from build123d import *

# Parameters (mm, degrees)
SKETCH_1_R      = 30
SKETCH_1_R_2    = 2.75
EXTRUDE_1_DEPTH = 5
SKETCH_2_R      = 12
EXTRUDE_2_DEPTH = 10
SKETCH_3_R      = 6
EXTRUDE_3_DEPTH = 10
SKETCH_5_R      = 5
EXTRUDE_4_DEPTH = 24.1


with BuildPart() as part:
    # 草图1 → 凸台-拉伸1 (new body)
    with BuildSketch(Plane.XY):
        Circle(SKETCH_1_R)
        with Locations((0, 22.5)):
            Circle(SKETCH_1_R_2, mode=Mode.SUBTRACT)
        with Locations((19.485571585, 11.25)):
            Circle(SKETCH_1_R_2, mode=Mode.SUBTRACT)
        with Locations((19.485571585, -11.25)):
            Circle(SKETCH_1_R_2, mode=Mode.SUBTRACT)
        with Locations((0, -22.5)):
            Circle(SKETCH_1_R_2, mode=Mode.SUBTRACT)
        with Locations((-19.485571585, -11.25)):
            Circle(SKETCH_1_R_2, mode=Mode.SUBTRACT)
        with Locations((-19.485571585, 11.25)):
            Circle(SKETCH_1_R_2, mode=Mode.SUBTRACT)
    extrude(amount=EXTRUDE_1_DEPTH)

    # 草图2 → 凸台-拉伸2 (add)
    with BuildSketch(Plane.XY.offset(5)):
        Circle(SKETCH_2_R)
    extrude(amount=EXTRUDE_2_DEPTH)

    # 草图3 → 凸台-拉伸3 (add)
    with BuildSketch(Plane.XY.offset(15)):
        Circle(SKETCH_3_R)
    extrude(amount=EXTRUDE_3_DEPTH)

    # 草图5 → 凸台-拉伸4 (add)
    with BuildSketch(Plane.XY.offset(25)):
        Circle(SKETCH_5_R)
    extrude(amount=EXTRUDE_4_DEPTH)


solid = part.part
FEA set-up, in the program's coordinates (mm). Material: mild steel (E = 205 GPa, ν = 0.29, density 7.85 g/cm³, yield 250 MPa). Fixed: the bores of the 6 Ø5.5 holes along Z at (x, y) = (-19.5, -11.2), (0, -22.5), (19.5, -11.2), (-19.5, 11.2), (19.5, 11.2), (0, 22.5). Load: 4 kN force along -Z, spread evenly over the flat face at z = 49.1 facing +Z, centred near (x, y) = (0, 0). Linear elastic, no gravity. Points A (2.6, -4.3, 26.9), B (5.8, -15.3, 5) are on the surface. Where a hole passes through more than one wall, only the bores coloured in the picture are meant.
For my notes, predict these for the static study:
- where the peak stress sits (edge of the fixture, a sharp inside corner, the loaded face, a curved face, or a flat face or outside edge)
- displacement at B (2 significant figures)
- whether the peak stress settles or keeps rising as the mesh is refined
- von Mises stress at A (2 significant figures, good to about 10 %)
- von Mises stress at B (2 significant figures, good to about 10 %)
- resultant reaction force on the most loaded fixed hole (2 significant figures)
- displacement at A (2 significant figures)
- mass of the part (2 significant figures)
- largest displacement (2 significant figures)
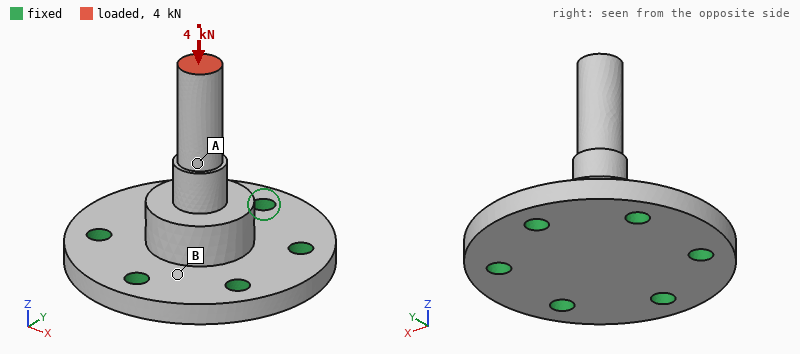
edge of the fixture
2.0 µm
keeps rising
52 MPa
13 MPa
730 N
7.5 µm
160 g
13 µm
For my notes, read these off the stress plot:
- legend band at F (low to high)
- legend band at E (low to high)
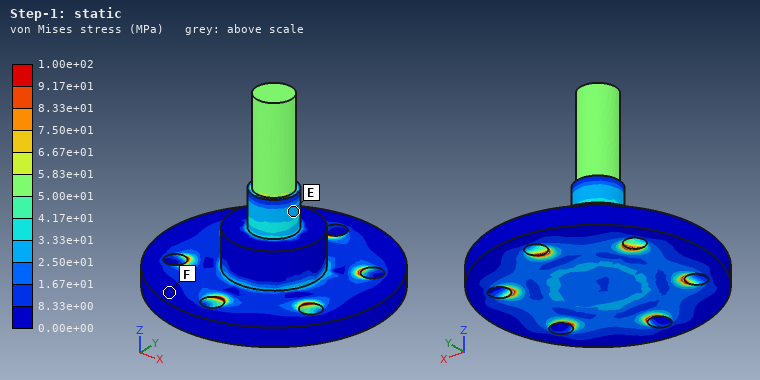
0.00e+00 to 8.33e+00 MPa
2.50e+01 to 3.33e+01 MPa
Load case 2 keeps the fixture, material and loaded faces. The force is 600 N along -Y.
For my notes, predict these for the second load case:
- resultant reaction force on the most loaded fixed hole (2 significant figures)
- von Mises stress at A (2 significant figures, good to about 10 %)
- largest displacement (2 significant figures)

560 N
110 MPa
79 µm
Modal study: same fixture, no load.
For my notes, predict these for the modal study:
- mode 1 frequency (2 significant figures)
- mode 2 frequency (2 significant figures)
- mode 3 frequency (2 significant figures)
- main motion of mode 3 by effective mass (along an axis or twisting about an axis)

5800 Hz
5800 Hz
16 kHz
along Z
